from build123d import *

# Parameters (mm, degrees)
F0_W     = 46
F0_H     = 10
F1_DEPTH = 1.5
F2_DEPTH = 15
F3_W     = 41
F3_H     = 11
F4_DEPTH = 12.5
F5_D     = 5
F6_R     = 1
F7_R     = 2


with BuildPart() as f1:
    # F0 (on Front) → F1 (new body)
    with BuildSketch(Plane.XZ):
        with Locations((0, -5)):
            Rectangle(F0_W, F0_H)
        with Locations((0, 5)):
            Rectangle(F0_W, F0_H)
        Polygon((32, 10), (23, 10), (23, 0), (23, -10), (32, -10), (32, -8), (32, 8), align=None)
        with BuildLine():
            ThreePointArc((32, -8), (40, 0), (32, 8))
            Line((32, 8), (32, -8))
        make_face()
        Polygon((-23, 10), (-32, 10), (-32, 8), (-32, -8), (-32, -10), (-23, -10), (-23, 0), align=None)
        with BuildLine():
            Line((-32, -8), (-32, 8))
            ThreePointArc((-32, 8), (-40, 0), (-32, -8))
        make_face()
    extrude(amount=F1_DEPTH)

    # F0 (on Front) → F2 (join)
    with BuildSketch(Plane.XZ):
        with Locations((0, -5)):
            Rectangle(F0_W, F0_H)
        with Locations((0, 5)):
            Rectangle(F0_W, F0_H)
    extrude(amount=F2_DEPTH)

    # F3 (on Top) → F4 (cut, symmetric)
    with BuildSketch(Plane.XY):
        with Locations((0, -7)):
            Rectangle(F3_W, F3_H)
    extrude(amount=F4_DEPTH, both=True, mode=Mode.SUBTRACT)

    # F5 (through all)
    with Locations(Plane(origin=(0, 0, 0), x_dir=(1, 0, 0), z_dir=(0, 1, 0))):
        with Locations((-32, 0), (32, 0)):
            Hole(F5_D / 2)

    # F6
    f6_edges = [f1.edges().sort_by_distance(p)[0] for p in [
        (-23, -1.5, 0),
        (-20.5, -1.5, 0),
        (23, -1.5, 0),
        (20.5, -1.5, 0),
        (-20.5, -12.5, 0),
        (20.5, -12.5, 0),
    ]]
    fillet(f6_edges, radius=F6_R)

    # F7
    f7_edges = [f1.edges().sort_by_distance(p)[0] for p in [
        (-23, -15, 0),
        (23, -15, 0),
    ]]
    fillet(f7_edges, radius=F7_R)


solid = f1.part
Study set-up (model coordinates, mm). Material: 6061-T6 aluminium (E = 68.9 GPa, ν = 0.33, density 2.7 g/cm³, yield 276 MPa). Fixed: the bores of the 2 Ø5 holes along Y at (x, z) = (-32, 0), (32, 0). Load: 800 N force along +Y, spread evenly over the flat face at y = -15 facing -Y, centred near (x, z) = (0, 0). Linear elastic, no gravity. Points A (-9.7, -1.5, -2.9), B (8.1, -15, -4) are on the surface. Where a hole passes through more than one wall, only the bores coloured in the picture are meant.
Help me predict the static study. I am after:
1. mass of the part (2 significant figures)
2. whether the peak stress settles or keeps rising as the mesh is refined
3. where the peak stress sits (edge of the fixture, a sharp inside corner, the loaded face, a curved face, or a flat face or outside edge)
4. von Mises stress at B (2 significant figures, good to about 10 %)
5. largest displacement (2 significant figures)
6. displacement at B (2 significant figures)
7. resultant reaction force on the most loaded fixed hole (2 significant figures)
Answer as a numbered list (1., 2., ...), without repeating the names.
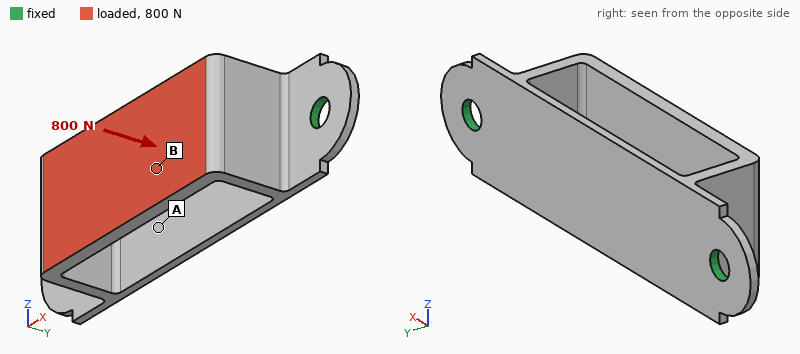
1. 15 g
2. keeps rising
3. edge of the fixture
4. 54 MPa
5. 0.19 mm
6. 0.15 mm
7. 490 N
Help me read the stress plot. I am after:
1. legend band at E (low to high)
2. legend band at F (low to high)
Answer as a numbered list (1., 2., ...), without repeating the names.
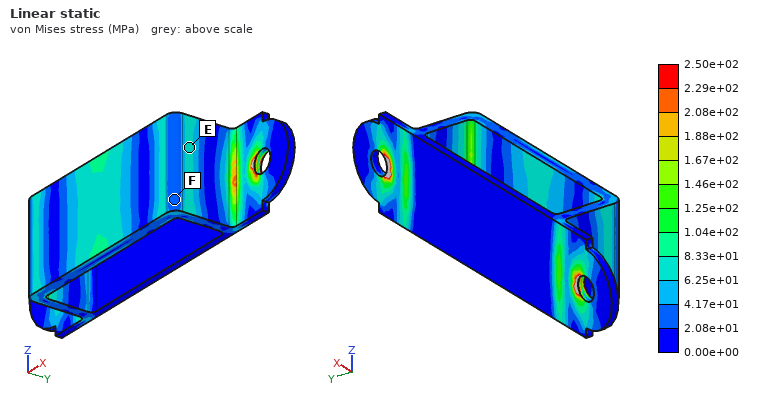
1. 6.25e+01 to 8.33e+01 MPa
2. 2.08e+01 to 4.17e+01 MPa
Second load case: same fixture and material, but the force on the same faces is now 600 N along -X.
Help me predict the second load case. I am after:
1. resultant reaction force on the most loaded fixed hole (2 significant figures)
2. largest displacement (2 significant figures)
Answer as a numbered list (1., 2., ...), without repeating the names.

1. 330 N
2. 0.13 mm
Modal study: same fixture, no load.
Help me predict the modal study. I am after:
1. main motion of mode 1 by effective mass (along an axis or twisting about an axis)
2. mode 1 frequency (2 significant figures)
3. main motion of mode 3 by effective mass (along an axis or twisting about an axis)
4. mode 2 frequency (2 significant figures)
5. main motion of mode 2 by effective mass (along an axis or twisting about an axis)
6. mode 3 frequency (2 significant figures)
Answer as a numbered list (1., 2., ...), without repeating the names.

1. along Z
2. 2000 Hz
3. along X
4. 3500 Hz
5. along Y
6. 3800 Hz
